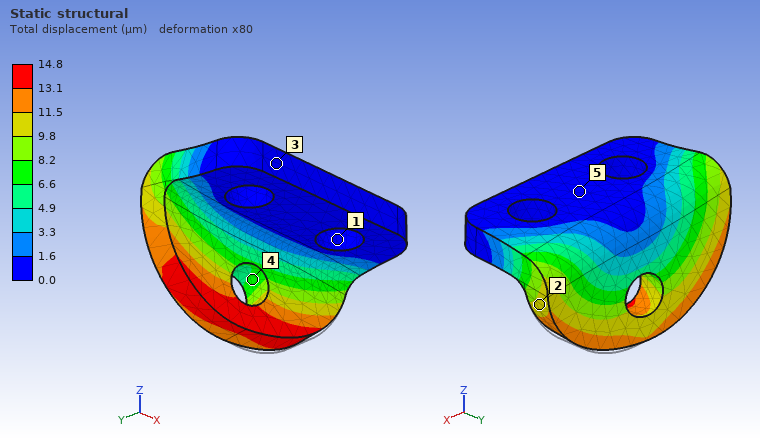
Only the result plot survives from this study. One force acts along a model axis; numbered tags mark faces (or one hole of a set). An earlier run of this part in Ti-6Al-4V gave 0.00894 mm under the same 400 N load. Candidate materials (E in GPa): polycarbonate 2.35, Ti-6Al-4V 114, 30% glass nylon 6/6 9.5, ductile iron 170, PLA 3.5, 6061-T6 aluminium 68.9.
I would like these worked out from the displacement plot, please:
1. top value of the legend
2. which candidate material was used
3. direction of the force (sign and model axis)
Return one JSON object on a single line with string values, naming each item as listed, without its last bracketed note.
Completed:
{"top value of the legend": "14.8 µm", "which candidate material was used": "6061-T6 aluminium", "direction of the force": "-X"}
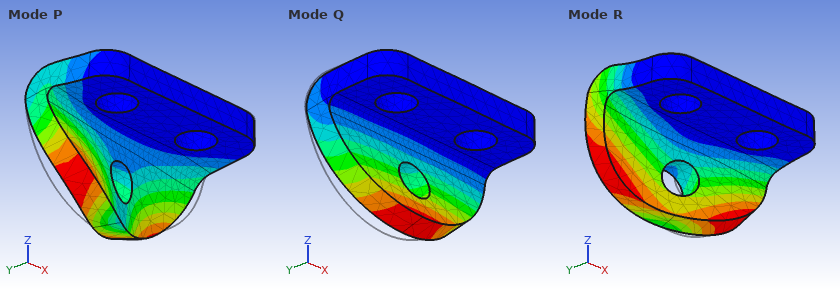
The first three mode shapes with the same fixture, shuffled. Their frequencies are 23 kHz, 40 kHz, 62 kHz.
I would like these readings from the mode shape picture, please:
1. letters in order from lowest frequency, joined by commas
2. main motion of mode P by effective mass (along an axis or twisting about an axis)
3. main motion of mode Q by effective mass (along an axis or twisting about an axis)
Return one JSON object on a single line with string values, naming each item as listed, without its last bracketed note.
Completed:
{"letters in order from lowest frequency, joined by commas": "Q, R, P", "main motion of mode P by effective mass": "along X", "main motion of mode Q by effective mass": "along Y"}
